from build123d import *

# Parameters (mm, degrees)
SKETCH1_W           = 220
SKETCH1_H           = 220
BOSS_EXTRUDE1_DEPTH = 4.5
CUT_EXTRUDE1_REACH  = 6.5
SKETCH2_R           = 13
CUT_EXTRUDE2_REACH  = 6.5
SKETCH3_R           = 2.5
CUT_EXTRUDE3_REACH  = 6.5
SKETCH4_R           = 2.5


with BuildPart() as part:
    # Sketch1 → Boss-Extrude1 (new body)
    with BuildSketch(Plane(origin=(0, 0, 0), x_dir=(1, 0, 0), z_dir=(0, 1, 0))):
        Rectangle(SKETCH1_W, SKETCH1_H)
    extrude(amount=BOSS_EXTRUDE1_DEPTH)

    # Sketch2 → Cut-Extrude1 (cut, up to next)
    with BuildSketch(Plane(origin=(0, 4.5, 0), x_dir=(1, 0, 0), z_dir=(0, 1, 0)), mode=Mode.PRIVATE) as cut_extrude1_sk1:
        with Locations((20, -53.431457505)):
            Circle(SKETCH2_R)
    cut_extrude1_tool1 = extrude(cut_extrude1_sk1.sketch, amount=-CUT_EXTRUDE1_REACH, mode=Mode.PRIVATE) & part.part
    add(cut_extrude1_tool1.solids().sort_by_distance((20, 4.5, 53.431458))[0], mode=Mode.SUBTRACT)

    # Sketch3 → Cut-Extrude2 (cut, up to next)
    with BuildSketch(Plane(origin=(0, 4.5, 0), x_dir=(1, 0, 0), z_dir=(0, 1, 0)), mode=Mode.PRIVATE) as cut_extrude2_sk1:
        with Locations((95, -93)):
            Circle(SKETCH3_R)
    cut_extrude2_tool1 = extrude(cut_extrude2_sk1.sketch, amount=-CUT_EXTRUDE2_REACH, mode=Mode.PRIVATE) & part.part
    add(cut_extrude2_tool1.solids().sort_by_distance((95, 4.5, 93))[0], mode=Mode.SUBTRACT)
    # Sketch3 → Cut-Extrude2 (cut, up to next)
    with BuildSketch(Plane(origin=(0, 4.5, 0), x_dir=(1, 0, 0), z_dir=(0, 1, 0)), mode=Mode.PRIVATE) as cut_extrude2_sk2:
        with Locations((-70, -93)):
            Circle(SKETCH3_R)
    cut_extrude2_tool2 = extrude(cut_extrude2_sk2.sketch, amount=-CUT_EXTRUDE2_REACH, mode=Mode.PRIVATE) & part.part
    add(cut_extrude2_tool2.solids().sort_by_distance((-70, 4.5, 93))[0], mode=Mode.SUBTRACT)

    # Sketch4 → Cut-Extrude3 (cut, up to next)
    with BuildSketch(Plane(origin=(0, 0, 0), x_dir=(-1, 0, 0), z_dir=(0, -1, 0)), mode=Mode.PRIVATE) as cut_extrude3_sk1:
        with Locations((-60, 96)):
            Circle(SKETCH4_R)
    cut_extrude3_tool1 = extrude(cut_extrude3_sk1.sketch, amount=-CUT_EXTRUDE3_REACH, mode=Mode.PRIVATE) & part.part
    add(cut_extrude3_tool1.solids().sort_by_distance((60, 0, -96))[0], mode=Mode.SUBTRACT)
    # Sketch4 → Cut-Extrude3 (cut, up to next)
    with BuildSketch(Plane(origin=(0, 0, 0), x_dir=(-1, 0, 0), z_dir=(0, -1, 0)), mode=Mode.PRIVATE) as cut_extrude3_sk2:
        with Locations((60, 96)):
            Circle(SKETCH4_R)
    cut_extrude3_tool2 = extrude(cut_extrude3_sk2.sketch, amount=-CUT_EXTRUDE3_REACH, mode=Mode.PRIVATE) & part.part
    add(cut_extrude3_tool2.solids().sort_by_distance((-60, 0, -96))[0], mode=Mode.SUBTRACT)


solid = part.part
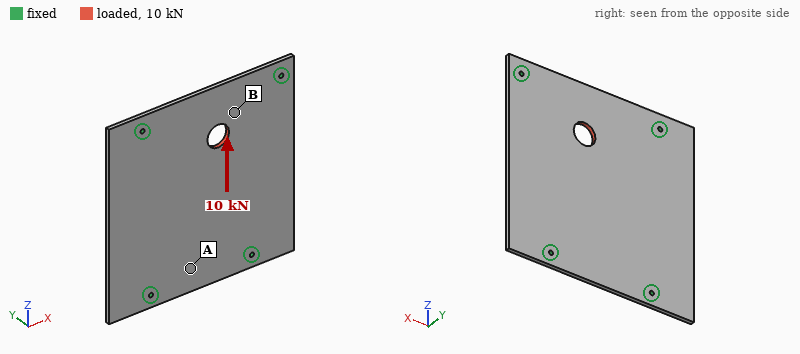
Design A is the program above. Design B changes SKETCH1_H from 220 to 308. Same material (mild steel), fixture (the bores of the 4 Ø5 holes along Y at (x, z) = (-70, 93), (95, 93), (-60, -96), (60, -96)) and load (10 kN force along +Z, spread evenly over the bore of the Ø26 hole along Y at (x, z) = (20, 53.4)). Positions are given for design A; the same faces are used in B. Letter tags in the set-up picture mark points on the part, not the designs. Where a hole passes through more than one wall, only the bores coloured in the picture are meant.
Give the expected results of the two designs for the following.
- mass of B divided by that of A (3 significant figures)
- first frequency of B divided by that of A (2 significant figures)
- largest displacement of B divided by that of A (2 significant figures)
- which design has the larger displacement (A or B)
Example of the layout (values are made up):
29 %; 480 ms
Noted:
1.41; 0.98; 0.76; A
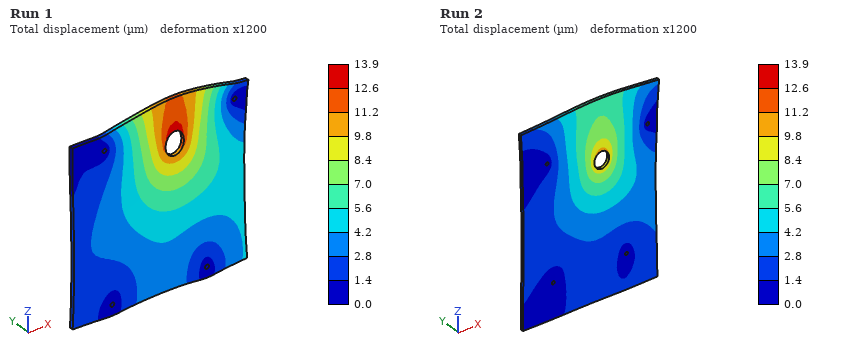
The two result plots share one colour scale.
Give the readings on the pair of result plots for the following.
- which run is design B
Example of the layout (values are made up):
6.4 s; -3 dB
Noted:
Run 2
